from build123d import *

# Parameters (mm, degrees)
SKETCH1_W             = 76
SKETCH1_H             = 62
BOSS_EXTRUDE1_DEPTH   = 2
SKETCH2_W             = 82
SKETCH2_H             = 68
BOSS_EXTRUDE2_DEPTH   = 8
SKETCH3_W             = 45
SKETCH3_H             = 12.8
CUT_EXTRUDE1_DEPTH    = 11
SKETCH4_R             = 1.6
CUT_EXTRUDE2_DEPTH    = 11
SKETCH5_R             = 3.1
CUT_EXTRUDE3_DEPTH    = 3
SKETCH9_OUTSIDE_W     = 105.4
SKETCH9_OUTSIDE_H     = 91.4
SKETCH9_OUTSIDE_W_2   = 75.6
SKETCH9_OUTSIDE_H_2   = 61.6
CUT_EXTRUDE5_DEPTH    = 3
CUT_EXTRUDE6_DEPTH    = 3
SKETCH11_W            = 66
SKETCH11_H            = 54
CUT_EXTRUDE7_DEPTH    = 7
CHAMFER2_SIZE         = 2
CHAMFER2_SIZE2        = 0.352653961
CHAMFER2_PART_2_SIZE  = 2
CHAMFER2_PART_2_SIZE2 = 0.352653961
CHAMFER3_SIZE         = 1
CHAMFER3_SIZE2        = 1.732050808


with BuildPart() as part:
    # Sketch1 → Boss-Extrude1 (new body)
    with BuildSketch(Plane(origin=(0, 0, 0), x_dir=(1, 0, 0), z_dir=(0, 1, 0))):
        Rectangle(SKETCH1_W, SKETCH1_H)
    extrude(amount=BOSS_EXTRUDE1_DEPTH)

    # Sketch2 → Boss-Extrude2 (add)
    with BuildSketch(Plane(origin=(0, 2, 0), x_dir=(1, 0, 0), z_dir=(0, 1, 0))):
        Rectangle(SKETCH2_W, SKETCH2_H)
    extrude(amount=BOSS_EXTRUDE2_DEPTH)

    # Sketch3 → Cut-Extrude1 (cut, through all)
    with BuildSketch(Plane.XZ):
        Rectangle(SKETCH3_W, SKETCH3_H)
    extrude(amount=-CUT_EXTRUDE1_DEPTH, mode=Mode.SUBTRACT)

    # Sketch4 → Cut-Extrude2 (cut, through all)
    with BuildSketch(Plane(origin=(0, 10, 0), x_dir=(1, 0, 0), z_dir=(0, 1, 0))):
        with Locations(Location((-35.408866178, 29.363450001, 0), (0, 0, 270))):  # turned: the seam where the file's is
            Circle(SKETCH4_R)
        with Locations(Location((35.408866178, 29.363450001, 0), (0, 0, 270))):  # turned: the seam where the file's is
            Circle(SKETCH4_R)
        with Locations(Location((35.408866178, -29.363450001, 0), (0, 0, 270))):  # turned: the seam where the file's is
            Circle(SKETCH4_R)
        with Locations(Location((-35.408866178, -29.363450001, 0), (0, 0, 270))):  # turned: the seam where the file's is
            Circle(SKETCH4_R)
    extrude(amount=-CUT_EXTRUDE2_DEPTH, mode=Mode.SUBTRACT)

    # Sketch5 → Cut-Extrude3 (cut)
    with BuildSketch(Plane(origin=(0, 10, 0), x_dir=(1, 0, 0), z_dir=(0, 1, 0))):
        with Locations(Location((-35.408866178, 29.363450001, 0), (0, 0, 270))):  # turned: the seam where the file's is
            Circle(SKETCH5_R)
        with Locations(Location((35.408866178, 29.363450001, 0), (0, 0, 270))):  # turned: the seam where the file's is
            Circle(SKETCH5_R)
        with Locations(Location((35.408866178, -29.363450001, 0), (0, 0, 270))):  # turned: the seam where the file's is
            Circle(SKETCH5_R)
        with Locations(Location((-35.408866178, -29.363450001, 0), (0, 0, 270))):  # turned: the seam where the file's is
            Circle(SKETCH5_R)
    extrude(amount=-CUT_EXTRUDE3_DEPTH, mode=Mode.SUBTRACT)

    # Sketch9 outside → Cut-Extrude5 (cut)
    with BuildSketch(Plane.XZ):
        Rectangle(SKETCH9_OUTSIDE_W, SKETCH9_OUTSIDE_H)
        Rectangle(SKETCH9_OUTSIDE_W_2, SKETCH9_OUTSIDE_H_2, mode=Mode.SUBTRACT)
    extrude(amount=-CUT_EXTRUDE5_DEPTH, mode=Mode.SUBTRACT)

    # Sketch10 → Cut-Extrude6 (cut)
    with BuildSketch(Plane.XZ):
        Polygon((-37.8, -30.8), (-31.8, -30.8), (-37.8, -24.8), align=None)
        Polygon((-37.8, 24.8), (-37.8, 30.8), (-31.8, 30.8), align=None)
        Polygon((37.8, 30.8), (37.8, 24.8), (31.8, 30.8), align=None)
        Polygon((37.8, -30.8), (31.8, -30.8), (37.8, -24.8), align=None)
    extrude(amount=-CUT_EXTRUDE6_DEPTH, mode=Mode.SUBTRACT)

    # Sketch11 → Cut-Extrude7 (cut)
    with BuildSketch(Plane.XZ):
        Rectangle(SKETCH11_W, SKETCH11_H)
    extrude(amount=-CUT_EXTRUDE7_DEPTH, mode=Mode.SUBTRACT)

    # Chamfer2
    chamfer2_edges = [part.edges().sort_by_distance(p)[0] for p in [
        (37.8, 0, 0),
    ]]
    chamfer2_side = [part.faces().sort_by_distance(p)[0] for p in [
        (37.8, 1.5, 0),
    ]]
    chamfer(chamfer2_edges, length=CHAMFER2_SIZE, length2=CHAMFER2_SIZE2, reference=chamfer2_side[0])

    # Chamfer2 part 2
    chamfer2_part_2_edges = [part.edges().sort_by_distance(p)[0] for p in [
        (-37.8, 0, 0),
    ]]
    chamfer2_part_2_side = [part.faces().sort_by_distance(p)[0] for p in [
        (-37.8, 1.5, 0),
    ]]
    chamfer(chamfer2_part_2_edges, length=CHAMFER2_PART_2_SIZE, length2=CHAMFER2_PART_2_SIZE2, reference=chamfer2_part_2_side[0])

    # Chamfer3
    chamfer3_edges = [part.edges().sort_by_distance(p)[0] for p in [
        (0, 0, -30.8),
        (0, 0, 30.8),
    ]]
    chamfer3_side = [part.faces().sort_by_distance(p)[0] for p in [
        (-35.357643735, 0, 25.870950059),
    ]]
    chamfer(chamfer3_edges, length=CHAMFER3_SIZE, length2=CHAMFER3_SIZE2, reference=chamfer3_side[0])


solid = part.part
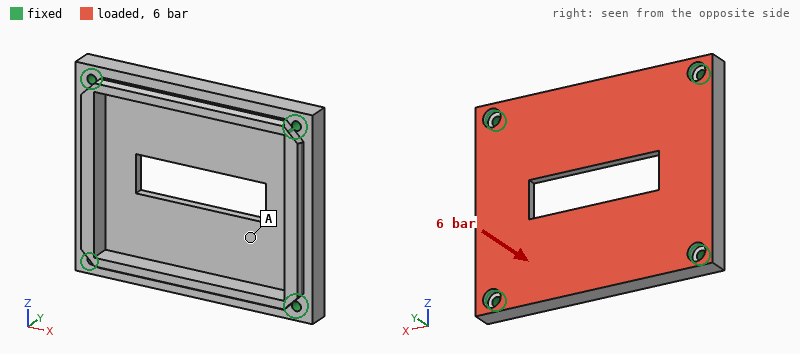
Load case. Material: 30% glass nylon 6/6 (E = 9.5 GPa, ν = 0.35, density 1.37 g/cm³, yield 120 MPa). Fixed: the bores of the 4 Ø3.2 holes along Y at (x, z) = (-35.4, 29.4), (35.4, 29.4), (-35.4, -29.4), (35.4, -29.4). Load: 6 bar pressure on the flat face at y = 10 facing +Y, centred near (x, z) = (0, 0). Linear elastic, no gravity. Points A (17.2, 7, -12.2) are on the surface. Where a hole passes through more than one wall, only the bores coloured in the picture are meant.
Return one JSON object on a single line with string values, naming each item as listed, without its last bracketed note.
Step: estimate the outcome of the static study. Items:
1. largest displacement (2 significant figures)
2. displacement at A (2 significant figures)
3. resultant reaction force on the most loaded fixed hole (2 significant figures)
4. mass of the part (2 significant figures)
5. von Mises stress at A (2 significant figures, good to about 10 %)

{"largest displacement": "1.2 mm", "displacement at A": "0.66 mm", "resultant reaction force on the most loaded fixed hole": "970 N", "mass of the part": "35 g", "von Mises stress at A": "25 MPa"}
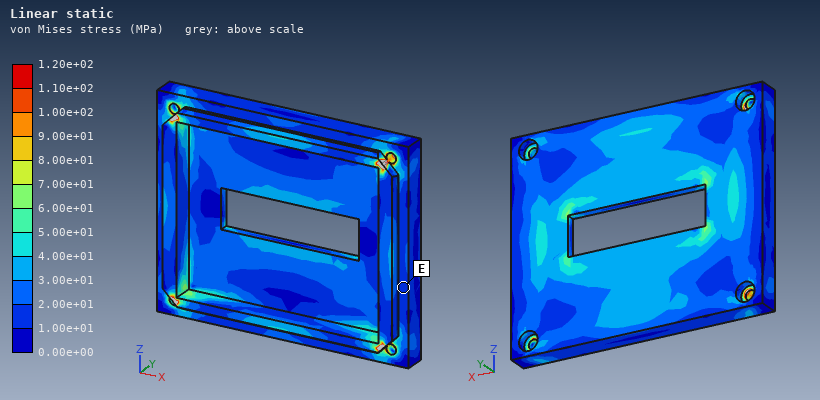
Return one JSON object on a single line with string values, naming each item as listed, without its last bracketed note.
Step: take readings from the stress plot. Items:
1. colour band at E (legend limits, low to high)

{"colour band at E": "1.00e+01 to 2.00e+01 MPa"}
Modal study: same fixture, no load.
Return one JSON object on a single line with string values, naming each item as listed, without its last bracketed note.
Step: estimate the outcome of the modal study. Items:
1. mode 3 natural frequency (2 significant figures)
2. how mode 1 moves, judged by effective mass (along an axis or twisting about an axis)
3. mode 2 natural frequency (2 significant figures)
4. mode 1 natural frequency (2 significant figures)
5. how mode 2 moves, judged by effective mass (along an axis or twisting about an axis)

{"mode 3 natural frequency": "4200 Hz", "how mode 1 moves, judged by effective mass": "along Y", "mode 2 natural frequency": "2800 Hz", "mode 1 natural frequency": "2300 Hz", "how mode 2 moves, judged by effective mass": "twisting about X"}
